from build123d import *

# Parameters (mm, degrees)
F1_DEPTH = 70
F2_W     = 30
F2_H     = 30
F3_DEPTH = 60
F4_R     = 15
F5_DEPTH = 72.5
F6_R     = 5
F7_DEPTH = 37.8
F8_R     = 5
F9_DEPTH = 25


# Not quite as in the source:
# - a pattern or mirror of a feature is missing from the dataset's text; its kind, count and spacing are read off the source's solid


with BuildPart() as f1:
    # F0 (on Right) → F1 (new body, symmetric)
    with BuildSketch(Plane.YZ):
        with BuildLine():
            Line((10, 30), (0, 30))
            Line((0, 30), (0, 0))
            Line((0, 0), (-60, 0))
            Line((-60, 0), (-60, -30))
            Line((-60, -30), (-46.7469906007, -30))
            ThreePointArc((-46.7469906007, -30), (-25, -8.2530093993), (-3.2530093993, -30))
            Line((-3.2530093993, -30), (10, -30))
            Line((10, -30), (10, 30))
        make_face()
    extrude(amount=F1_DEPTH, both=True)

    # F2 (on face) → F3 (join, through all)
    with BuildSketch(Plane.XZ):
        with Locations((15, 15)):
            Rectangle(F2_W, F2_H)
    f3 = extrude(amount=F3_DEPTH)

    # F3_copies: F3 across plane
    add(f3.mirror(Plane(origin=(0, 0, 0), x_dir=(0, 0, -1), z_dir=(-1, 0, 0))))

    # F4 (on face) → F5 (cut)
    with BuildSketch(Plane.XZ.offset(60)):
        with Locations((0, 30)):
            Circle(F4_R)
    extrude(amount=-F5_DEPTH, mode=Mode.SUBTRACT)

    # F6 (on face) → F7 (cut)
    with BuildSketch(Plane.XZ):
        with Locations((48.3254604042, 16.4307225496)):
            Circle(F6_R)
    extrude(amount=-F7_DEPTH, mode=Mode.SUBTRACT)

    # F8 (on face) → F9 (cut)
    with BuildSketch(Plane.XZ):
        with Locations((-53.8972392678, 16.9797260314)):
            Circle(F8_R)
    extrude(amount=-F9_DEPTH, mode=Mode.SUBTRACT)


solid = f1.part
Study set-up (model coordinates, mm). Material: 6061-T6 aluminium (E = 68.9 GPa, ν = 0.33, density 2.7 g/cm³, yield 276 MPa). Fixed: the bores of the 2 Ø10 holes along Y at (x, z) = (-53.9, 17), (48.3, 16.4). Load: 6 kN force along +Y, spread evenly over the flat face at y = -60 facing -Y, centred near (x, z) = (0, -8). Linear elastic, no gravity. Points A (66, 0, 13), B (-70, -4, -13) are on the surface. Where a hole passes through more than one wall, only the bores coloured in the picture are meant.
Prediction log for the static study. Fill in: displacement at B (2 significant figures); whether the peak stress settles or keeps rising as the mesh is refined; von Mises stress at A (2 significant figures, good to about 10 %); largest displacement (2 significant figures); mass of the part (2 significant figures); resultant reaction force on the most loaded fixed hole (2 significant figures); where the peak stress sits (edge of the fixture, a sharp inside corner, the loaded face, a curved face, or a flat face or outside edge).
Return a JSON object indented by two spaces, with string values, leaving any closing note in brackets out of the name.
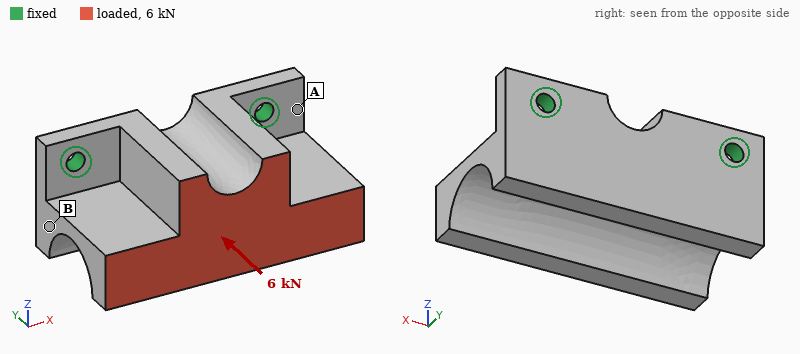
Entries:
{
  "displacement at B": "0.066 mm",
  "whether the peak stress settles or keeps rising as the mesh is refined": "keeps rising",
  "von Mises stress at A": "30 MPa",
  "largest displacement": "0.19 mm",
  "mass of the part": "850 g",
  "resultant reaction force on the most loaded fixed hole": "3.1 kN",
  "where the peak stress sits": "edge of the fixture"
}
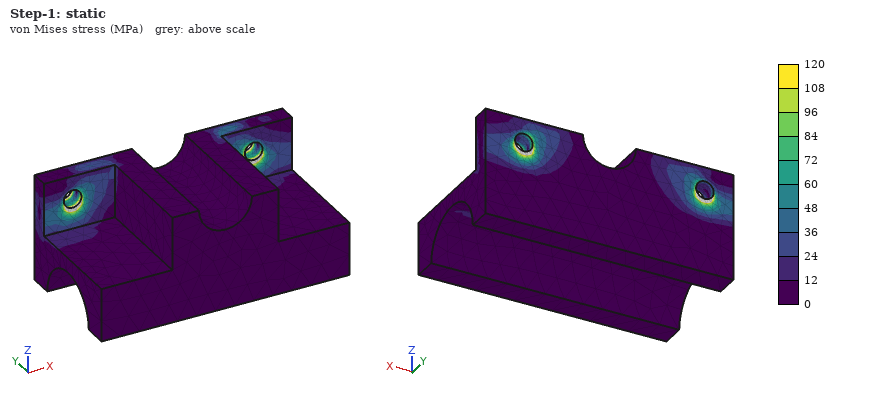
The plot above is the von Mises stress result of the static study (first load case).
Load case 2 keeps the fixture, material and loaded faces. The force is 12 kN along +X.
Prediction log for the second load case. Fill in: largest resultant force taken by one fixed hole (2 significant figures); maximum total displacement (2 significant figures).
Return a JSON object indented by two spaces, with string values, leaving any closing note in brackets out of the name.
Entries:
{
  "largest resultant force taken by one fixed hole": "10 kN",
  "maximum total displacement": "96 µm"
}
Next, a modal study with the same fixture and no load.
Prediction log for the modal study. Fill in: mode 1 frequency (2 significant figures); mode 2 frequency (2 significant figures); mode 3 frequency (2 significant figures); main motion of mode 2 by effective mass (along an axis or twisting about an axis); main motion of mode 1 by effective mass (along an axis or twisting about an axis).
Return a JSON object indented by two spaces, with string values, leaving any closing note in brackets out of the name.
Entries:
{
  "mode 1 frequency": "900 Hz",
  "mode 2 frequency": "3100 Hz",
  "mode 3 frequency": "3600 Hz",
  "main motion of mode 2 by effective mass": "along X",
  "main motion of mode 1 by effective mass": "along Z"
}
